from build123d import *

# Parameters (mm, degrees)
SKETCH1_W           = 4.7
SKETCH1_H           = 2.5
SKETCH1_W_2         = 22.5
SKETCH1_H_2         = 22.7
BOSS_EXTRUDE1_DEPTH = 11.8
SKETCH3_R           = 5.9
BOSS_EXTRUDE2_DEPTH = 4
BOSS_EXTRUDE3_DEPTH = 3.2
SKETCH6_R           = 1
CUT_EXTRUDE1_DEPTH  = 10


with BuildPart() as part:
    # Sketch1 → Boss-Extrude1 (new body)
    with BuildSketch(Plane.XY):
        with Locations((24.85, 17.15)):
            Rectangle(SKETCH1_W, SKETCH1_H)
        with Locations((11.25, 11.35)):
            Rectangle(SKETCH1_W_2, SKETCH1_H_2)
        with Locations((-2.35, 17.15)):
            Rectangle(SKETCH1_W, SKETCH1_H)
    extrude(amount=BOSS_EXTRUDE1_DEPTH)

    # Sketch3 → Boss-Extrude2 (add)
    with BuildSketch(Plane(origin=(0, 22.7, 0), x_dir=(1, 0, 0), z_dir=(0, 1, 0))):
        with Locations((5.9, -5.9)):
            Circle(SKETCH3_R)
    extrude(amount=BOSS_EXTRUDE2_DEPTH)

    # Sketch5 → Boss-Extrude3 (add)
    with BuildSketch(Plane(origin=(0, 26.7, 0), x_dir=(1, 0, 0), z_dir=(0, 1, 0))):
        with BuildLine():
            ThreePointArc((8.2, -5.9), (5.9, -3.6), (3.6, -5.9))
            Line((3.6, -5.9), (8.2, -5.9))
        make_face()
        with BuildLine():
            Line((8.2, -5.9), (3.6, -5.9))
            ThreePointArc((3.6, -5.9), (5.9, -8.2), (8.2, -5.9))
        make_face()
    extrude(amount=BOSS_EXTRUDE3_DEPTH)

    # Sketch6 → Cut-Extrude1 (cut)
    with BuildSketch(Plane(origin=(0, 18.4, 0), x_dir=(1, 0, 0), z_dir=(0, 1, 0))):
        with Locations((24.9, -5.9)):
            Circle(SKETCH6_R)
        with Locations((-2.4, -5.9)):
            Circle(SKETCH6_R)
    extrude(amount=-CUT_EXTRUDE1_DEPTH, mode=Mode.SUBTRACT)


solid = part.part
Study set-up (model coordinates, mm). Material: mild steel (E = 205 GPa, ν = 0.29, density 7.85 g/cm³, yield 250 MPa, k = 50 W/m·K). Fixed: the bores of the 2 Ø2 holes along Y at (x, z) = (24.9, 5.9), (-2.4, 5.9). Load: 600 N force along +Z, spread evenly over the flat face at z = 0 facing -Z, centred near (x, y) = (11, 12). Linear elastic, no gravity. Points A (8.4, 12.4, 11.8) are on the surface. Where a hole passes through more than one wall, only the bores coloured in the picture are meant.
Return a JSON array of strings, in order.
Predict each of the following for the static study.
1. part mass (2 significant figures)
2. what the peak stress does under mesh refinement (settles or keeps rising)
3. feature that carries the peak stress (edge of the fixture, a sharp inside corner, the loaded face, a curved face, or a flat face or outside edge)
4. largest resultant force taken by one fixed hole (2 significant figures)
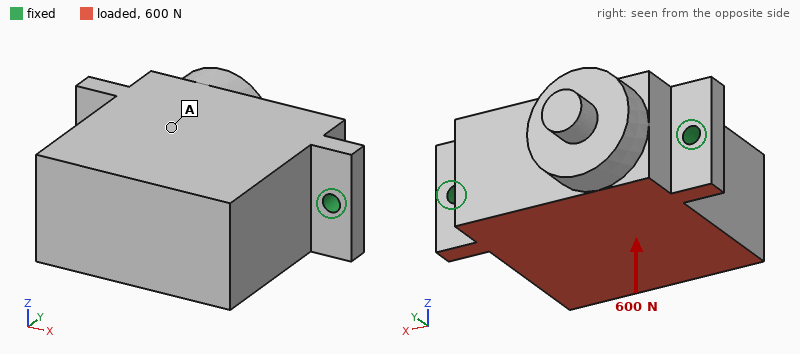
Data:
["53 g", "keeps rising", "edge of the fixture", "300 N"]
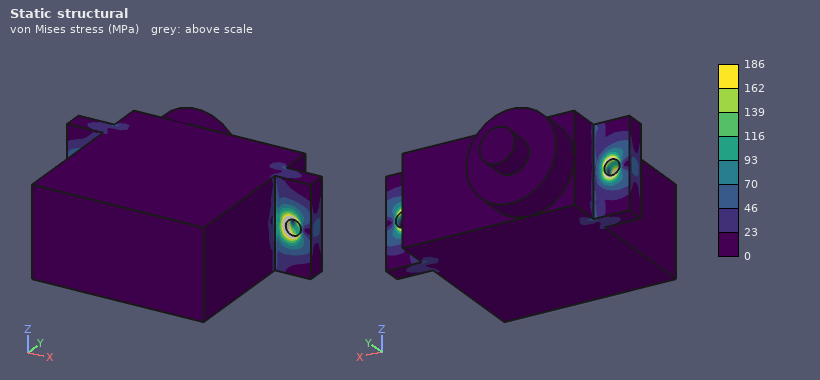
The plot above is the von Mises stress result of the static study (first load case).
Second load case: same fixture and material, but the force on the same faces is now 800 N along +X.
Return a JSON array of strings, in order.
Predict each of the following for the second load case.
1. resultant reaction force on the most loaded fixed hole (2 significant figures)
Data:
["470 N"]
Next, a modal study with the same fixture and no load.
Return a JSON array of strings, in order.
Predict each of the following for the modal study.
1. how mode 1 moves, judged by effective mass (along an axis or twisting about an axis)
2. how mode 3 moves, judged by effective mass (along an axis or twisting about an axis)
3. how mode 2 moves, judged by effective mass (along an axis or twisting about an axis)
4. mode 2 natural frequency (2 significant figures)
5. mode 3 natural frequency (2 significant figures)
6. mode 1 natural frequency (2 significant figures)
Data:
["along Z", "along X", "along Y", "16 kHz", "17 kHz", "4000 Hz"]
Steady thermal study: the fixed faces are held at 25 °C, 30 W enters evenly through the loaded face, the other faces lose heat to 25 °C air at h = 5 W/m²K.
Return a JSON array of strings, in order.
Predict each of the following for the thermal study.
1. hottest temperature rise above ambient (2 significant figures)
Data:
["67 K"]
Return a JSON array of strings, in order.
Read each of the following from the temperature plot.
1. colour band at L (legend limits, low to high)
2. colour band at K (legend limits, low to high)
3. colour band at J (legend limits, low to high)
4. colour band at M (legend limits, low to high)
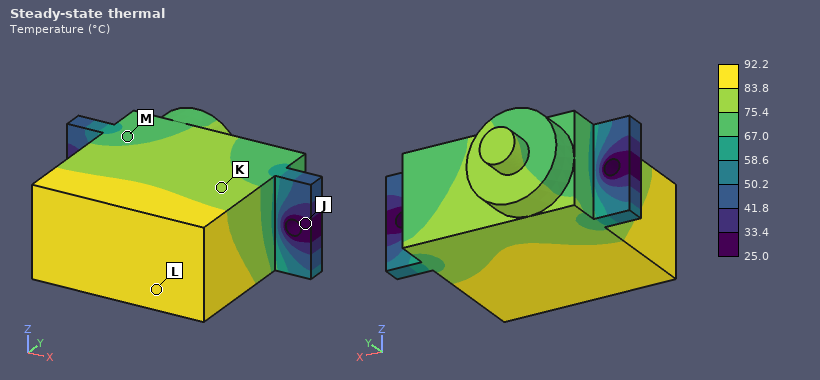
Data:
["83.8 to 92.2 °C", "75.4 to 83.8 °C", "25.0 to 33.4 °C", "67.0 to 75.4 °C"]
